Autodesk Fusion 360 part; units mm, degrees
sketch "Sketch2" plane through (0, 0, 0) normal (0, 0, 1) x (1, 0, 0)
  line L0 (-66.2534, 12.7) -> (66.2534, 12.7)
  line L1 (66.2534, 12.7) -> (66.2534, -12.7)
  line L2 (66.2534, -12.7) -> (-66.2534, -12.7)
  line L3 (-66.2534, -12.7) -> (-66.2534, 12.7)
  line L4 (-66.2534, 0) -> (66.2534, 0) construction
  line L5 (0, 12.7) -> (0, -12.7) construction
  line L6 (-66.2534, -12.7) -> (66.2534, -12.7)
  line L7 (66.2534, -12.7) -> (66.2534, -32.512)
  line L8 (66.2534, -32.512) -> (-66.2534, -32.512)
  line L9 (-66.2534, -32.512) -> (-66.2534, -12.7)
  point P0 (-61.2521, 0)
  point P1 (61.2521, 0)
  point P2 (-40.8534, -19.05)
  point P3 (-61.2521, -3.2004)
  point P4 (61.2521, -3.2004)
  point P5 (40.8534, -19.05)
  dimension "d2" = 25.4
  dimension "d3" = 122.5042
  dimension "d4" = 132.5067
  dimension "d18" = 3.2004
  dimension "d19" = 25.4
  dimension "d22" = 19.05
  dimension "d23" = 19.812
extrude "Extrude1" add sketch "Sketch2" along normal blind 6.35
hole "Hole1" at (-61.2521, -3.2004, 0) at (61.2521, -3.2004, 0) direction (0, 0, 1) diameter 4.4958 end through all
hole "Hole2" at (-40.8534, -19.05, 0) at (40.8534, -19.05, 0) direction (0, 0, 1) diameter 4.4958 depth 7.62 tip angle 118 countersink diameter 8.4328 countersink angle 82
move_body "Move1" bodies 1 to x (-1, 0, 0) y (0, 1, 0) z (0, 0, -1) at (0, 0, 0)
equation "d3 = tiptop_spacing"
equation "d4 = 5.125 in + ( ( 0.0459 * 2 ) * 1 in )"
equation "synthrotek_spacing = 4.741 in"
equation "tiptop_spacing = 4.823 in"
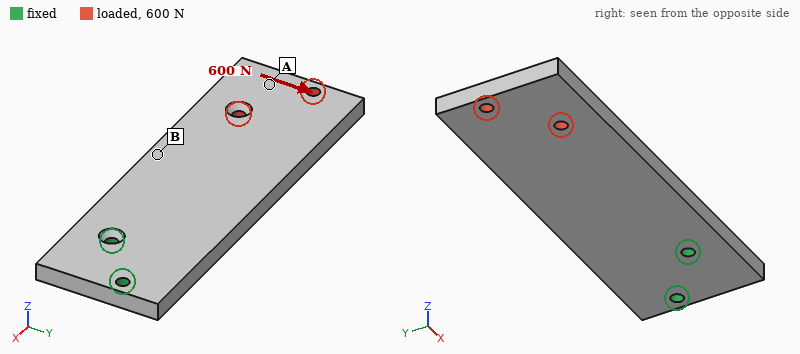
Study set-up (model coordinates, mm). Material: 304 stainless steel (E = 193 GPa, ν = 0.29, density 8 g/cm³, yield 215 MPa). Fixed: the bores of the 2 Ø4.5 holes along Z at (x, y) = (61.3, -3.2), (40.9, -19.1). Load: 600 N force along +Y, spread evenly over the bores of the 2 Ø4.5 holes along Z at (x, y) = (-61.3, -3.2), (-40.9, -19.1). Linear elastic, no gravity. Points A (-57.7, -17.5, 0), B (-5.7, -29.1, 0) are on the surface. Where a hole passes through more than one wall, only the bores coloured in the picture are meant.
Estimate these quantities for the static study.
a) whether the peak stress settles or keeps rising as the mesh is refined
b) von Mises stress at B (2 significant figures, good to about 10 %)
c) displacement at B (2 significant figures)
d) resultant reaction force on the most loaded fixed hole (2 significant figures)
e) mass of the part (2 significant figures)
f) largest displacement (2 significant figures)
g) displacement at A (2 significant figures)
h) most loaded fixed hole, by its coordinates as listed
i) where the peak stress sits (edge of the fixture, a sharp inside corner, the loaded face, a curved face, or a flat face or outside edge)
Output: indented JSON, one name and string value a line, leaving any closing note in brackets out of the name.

{
  "whether the peak stress settles or keeps rising as the mesh is refined": "keeps rising",
  "von Mises stress at B": "11 MPa",
  "displacement at B": "16 µm",
  "resultant reaction force on the most loaded fixed hole": "2.4 kN",
  "mass of the part": "300 g",
  "largest displacement": "43 µm",
  "displacement at A": "38 µm",
  "most loaded fixed hole, by its coordinates as listed": "(40.9, -19.1)",
  "where the peak stress sits": "edge of the fixture"
}
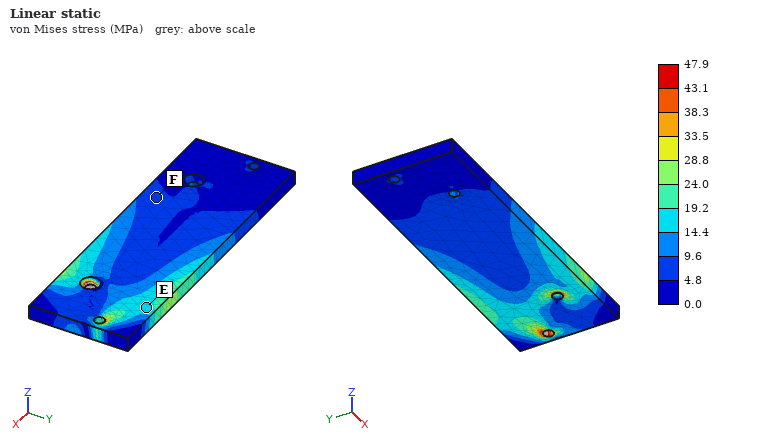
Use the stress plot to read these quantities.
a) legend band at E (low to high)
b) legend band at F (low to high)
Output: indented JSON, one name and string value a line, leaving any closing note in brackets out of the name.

{
  "legend band at E": "14.4 to 19.2 MPa",
  "legend band at F": "4.8 to 9.6 MPa"
}
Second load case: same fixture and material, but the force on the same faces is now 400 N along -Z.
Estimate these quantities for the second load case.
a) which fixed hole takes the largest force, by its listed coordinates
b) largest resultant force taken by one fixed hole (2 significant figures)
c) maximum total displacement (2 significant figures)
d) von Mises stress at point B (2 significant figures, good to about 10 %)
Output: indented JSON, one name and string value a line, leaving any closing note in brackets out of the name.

{
  "which fixed hole takes the largest force, by its listed coordinates": "(40.9, -19.1)",
  "largest resultant force taken by one fixed hole": "1.2 kN",
  "maximum total displacement": "0.89 mm",
  "von Mises stress at point B": "63 MPa"
}
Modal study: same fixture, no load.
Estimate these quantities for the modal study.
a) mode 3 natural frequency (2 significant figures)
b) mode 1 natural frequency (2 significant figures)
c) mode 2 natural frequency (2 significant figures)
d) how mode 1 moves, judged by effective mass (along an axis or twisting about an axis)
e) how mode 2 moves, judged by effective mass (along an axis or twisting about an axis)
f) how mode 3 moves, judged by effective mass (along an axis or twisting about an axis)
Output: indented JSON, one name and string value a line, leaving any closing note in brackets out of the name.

{
  "mode 3 natural frequency": "2100 Hz",
  "mode 1 natural frequency": "400 Hz",
  "mode 2 natural frequency": "1800 Hz",
  "how mode 1 moves, judged by effective mass": "along Z",
  "how mode 2 moves, judged by effective mass": "twisting about X",
  "how mode 3 moves, judged by effective mass": "along Y"
}
